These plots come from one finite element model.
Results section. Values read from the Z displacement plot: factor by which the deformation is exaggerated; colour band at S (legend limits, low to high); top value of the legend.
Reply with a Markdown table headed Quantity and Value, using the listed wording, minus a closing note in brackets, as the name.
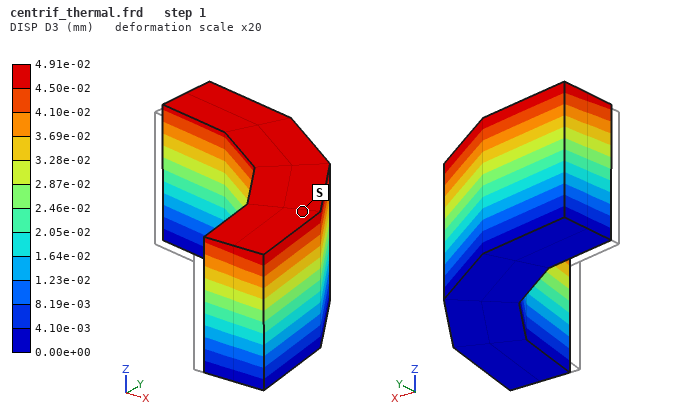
| Quantity | Value |
|---|---|
| factor by which the deformation is exaggerated | 20 |
| colour band at S | 4.50e-02 to 4.91e-02 mm |
| top value of the legend | 4.91e-02 mm |
